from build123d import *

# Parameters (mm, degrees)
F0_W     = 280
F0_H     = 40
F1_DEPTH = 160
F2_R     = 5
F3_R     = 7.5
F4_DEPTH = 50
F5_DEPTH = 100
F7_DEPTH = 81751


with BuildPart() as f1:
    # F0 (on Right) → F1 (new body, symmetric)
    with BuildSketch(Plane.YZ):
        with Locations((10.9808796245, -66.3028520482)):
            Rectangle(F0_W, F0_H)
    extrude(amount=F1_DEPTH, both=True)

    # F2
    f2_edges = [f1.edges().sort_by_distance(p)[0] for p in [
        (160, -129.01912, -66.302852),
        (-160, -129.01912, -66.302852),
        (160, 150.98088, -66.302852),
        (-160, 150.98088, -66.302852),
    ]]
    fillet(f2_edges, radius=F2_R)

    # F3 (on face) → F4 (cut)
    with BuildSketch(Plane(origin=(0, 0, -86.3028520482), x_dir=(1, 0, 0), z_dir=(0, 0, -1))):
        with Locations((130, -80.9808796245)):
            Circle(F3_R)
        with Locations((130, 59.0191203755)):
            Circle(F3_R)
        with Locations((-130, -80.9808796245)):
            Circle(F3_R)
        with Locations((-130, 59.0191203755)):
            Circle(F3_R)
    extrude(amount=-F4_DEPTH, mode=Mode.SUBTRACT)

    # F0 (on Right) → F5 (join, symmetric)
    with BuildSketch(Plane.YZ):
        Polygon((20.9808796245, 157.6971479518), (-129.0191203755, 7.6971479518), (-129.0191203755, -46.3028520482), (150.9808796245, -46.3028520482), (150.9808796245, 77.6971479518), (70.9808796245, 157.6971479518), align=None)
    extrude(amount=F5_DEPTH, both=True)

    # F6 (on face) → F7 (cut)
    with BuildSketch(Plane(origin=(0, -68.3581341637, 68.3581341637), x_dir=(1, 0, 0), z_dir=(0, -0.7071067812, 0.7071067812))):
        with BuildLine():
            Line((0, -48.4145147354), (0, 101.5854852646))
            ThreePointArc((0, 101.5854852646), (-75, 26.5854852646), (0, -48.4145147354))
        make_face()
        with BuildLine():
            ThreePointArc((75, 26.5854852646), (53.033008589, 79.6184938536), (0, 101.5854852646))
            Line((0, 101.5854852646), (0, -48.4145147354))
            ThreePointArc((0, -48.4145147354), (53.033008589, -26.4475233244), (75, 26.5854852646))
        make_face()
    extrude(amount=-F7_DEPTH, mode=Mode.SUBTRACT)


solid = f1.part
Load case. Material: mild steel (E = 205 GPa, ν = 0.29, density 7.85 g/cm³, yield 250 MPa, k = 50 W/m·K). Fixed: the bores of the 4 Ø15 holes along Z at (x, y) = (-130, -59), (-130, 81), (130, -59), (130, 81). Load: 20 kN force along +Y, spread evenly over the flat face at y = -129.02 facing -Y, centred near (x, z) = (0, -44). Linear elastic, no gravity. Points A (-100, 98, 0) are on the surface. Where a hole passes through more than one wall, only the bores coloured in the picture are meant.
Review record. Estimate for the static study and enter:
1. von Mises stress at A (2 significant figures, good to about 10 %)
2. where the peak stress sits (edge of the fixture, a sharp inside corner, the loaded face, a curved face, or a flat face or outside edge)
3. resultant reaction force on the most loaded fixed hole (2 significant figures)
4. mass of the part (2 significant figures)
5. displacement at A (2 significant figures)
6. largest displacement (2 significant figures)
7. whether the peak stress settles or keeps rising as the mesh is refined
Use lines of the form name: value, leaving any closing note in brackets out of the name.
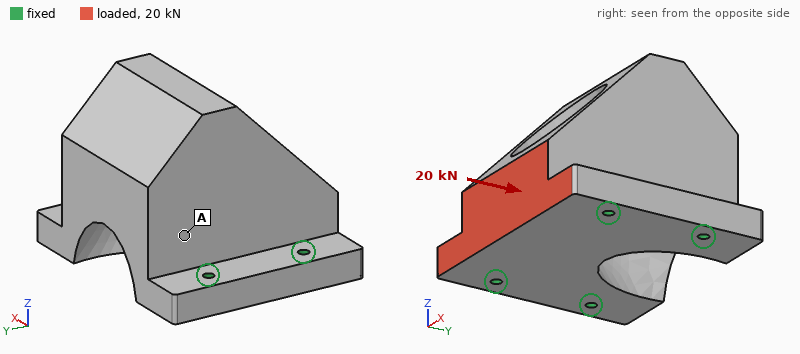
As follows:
von Mises stress at A: 0.48 MPa
where the peak stress sits: edge of the fixture
resultant reaction force on the most loaded fixed hole: 6.4 kN
mass of the part: 63 kg
displacement at A: 1.4 µm
largest displacement: 2.7 µm
whether the peak stress settles or keeps rising as the mesh is refined: keeps rising
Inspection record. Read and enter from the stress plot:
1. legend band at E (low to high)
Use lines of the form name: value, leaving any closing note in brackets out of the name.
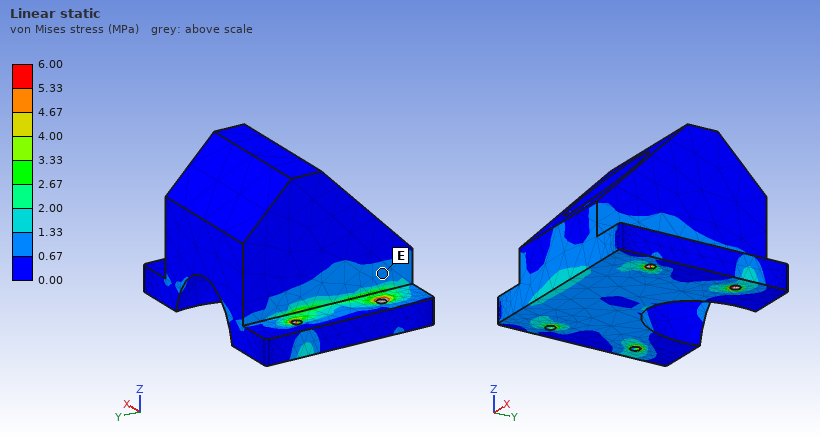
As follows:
legend band at E: 0.67 to 1.33 MPa
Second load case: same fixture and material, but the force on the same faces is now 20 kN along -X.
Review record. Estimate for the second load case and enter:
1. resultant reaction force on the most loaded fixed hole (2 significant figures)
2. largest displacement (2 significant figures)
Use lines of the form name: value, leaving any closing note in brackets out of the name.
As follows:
resultant reaction force on the most loaded fixed hole: 9.9 kN
largest displacement: 2.3 µm
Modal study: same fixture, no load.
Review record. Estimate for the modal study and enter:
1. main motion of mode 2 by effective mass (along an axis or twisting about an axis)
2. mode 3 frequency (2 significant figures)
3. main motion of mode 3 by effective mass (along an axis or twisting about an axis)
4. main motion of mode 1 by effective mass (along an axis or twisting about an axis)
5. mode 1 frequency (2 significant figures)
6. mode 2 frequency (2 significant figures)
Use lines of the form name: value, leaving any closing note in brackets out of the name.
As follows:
main motion of mode 2 by effective mass: along X
mode 3 frequency: 2100 Hz
main motion of mode 3 by effective mass: along Z
main motion of mode 1 by effective mass: along Y
mode 1 frequency: 1100 Hz
mode 2 frequency: 1400 Hz
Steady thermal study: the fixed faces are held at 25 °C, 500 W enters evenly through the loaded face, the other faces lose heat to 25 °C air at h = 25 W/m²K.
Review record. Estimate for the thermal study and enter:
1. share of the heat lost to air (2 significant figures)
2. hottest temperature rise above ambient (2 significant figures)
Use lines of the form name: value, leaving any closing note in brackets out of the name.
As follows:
share of the heat lost to air: 33 %
hottest temperature rise above ambient: 60 K
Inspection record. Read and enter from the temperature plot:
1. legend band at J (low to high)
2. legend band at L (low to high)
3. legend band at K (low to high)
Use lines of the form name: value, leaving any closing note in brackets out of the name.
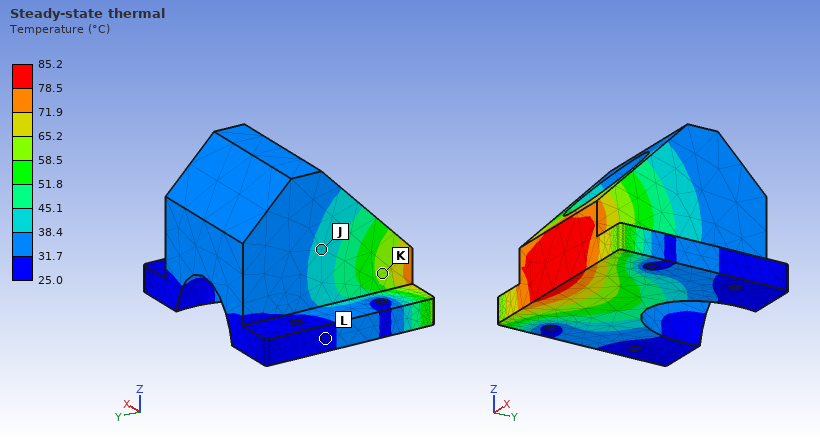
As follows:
legend band at J: 38.4 to 45.1 °C
legend band at L: 25.0 to 31.7 °C
legend band at K: 58.5 to 65.2 °C
